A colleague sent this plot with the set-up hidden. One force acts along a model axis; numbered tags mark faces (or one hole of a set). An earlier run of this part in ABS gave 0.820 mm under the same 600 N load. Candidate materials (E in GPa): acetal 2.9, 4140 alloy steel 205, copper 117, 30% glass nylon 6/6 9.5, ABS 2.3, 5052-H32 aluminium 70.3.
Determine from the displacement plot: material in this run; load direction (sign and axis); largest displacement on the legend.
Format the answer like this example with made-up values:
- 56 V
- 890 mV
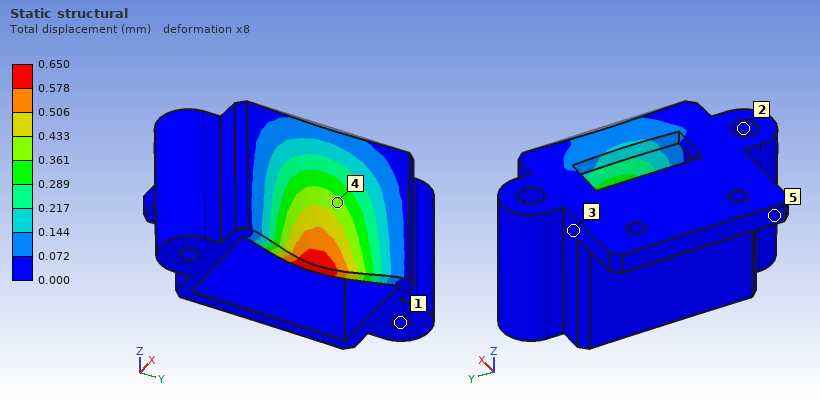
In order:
- acetal
- -X
- 0.650 mm
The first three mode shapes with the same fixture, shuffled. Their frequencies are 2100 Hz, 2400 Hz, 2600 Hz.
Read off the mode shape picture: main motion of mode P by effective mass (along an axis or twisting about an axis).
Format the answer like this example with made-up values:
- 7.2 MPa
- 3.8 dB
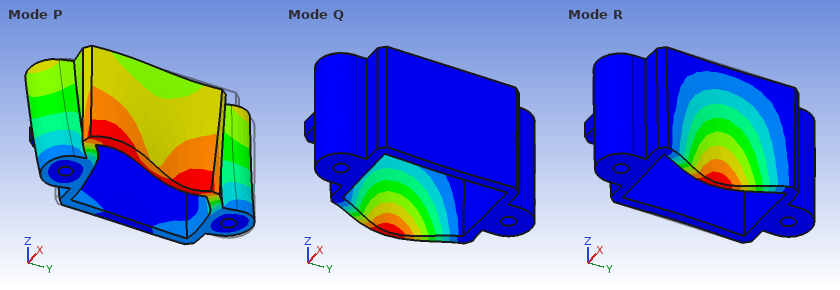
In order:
- along Y
